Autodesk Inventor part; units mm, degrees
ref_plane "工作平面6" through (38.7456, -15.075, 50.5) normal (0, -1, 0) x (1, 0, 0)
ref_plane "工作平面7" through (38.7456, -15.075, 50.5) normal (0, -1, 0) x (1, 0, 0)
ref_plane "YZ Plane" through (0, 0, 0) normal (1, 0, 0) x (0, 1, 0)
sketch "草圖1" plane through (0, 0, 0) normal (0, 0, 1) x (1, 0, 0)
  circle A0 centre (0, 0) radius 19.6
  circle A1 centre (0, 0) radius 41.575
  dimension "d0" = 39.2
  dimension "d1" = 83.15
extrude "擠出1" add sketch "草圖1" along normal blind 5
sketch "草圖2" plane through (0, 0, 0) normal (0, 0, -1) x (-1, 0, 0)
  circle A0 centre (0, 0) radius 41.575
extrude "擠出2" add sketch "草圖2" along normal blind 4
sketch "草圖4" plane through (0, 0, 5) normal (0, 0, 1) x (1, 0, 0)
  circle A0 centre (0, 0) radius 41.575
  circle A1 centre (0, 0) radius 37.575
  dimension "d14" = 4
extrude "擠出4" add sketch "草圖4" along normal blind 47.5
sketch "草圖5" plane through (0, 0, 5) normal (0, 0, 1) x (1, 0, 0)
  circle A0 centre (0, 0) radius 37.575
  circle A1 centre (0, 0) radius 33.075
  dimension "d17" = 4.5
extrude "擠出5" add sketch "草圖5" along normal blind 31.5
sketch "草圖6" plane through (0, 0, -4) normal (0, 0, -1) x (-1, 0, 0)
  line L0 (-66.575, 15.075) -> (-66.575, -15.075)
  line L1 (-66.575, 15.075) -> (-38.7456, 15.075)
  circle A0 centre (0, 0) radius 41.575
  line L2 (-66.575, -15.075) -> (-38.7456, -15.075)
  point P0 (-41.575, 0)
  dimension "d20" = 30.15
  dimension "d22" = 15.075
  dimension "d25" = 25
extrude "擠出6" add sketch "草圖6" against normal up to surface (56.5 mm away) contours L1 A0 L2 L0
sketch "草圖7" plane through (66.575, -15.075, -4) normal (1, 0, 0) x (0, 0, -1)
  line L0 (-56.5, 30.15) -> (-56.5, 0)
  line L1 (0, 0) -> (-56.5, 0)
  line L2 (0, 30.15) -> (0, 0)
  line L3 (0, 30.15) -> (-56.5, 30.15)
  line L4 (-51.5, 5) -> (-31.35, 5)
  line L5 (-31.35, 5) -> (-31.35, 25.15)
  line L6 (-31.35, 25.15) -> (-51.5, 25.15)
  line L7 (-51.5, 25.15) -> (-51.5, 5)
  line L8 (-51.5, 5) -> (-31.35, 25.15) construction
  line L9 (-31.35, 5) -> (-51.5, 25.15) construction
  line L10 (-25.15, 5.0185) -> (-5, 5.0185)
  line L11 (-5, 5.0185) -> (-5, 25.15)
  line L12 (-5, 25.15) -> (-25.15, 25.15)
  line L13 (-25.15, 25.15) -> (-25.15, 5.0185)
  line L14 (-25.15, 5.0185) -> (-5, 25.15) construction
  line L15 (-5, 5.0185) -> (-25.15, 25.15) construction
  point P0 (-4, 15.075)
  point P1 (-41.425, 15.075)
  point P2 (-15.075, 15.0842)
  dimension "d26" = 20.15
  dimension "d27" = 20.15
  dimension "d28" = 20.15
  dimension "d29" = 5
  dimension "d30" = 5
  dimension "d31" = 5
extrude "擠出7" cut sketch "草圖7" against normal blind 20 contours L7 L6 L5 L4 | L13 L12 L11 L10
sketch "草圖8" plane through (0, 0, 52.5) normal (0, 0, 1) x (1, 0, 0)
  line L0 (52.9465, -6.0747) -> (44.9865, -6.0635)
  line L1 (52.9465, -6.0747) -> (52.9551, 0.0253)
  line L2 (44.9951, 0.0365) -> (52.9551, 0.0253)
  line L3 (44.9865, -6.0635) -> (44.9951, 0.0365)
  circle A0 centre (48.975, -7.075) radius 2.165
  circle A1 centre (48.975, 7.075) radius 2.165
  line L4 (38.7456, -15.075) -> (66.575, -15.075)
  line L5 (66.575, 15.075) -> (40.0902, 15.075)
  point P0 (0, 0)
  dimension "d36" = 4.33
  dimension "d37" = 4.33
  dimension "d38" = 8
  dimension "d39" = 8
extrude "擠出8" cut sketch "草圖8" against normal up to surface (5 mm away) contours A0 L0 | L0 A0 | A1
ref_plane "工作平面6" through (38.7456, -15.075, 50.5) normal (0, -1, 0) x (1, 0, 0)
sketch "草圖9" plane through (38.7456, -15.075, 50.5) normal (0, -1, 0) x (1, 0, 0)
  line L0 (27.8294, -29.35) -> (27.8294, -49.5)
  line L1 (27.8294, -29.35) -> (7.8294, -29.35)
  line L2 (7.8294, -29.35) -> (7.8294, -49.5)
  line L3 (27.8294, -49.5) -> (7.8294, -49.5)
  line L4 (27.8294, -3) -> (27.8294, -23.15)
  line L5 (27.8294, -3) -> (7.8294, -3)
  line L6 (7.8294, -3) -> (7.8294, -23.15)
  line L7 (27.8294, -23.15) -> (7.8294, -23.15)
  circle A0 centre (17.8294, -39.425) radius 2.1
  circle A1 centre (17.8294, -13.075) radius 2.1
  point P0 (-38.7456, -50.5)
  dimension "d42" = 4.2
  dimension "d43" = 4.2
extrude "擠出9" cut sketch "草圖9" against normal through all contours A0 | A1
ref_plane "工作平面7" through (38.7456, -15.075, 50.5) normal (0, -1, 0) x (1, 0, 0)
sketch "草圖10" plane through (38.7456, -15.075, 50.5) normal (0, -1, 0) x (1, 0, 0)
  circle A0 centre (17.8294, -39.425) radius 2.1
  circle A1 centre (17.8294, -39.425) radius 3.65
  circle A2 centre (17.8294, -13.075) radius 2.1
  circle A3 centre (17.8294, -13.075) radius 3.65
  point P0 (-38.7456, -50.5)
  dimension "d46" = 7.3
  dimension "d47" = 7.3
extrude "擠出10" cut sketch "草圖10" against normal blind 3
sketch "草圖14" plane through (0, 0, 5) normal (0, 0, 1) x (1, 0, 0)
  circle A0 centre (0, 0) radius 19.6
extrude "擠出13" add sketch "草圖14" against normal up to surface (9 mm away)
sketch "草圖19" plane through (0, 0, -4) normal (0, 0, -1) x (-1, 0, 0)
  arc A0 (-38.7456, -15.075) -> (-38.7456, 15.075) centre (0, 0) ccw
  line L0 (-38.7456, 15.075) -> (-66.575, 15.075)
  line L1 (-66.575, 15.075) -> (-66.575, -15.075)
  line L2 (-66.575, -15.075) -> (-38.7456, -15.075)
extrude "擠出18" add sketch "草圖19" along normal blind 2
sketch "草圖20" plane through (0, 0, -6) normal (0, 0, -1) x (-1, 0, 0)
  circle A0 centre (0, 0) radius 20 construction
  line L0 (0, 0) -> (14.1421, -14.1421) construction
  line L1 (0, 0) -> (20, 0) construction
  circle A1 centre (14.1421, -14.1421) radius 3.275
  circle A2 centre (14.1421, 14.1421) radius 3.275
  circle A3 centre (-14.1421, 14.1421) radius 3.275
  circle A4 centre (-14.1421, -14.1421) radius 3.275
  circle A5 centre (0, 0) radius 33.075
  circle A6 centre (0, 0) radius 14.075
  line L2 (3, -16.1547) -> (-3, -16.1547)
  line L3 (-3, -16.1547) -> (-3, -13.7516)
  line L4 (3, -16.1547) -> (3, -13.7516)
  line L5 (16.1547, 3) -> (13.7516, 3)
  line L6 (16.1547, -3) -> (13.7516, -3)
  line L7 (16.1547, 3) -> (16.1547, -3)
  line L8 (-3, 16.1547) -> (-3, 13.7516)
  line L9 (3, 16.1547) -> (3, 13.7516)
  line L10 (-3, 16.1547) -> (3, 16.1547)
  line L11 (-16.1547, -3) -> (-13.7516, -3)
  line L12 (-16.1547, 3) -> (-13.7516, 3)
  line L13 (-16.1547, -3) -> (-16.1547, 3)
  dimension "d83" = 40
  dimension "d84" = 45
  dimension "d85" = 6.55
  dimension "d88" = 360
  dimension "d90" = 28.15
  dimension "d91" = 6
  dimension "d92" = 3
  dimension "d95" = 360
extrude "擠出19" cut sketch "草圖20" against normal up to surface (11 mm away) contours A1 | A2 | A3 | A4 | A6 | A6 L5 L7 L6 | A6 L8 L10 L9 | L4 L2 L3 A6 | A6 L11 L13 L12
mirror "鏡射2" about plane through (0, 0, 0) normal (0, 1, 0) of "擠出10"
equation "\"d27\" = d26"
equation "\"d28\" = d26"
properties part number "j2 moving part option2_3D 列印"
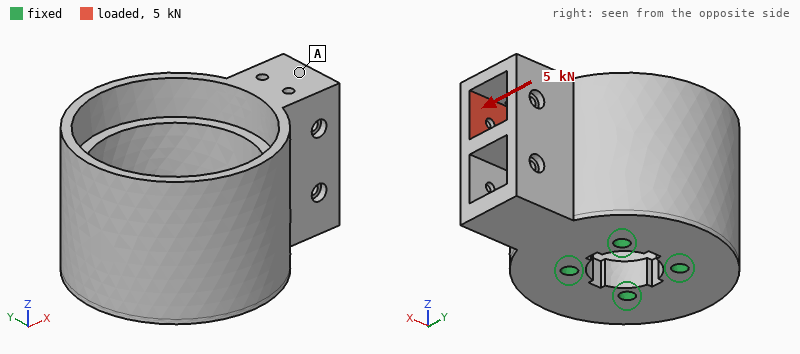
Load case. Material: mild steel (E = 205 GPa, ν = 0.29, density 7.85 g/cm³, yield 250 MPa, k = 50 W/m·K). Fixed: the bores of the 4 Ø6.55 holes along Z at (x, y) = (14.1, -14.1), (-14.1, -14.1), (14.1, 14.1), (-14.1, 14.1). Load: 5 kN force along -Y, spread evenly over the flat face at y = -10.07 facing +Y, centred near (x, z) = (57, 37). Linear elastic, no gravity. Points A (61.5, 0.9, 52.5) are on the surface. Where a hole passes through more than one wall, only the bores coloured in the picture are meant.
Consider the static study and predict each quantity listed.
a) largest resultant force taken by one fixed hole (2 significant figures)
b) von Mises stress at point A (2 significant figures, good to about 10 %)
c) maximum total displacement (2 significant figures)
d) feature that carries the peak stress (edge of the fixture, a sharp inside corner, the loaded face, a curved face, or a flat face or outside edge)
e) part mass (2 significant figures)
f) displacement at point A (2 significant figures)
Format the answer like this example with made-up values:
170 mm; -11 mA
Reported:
5.4 kN; 12 MPa; 37 µm; a curved face; 1.2 kg; 27 µm
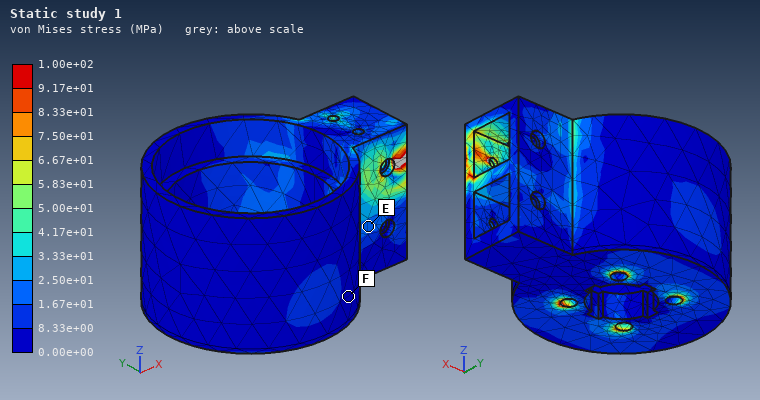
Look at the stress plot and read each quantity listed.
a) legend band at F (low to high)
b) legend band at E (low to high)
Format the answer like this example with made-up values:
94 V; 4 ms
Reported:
0.00e+00 to 8.33e+00 MPa; 1.67e+01 to 2.50e+01 MPa
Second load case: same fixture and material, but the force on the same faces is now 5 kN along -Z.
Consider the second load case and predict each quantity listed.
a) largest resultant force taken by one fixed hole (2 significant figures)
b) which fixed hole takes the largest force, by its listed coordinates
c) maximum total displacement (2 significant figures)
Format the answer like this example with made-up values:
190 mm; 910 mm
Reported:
5.2 kN; (14.1, -14.1); 65 µm
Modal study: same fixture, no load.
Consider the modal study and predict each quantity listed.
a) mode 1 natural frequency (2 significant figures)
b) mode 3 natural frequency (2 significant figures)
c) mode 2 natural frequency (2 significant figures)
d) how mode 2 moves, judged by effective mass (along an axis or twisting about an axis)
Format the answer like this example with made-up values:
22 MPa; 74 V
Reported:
3000 Hz; 4700 Hz; 4200 Hz; along Y
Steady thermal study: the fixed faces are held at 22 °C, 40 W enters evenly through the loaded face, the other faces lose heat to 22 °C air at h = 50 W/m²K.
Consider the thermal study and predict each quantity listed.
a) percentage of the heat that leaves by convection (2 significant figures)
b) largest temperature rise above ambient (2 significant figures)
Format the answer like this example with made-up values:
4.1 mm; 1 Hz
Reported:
52 %; 71 K
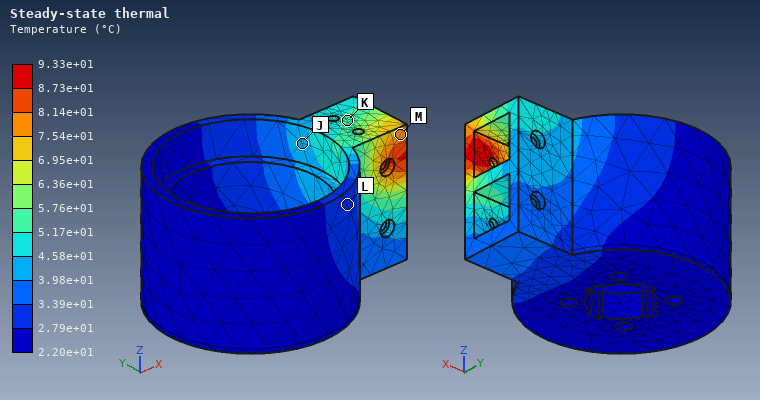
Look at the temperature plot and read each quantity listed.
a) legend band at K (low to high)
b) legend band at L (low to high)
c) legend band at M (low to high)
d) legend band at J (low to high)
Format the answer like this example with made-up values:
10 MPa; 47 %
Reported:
5.17e+01 to 5.76e+01 °C; 2.79e+01 to 3.39e+01 °C; 7.54e+01 to 8.14e+01 °C; 3.98e+01 to 4.58e+01 °C
